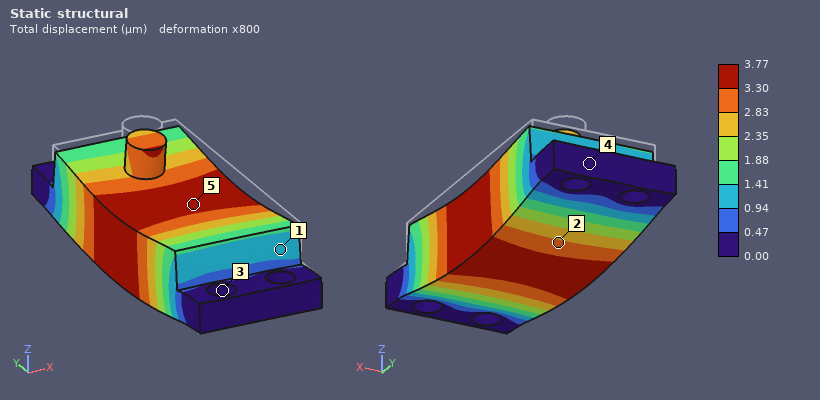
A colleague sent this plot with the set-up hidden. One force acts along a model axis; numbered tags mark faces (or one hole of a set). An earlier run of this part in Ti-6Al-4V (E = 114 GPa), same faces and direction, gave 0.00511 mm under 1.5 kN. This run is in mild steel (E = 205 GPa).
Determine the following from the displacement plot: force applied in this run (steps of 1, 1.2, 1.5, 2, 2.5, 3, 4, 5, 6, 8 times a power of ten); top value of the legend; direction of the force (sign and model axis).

2 kN
3.77 µm
-Z
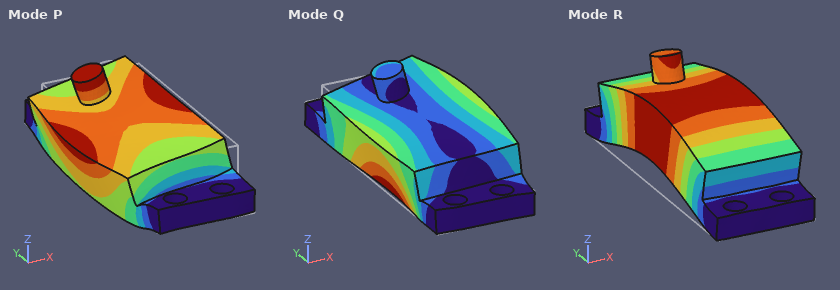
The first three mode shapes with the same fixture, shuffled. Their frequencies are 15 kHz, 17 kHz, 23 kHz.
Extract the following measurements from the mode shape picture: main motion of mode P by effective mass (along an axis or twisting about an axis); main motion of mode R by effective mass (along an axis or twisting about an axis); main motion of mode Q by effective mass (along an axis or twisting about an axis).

along X
along Z
along X
